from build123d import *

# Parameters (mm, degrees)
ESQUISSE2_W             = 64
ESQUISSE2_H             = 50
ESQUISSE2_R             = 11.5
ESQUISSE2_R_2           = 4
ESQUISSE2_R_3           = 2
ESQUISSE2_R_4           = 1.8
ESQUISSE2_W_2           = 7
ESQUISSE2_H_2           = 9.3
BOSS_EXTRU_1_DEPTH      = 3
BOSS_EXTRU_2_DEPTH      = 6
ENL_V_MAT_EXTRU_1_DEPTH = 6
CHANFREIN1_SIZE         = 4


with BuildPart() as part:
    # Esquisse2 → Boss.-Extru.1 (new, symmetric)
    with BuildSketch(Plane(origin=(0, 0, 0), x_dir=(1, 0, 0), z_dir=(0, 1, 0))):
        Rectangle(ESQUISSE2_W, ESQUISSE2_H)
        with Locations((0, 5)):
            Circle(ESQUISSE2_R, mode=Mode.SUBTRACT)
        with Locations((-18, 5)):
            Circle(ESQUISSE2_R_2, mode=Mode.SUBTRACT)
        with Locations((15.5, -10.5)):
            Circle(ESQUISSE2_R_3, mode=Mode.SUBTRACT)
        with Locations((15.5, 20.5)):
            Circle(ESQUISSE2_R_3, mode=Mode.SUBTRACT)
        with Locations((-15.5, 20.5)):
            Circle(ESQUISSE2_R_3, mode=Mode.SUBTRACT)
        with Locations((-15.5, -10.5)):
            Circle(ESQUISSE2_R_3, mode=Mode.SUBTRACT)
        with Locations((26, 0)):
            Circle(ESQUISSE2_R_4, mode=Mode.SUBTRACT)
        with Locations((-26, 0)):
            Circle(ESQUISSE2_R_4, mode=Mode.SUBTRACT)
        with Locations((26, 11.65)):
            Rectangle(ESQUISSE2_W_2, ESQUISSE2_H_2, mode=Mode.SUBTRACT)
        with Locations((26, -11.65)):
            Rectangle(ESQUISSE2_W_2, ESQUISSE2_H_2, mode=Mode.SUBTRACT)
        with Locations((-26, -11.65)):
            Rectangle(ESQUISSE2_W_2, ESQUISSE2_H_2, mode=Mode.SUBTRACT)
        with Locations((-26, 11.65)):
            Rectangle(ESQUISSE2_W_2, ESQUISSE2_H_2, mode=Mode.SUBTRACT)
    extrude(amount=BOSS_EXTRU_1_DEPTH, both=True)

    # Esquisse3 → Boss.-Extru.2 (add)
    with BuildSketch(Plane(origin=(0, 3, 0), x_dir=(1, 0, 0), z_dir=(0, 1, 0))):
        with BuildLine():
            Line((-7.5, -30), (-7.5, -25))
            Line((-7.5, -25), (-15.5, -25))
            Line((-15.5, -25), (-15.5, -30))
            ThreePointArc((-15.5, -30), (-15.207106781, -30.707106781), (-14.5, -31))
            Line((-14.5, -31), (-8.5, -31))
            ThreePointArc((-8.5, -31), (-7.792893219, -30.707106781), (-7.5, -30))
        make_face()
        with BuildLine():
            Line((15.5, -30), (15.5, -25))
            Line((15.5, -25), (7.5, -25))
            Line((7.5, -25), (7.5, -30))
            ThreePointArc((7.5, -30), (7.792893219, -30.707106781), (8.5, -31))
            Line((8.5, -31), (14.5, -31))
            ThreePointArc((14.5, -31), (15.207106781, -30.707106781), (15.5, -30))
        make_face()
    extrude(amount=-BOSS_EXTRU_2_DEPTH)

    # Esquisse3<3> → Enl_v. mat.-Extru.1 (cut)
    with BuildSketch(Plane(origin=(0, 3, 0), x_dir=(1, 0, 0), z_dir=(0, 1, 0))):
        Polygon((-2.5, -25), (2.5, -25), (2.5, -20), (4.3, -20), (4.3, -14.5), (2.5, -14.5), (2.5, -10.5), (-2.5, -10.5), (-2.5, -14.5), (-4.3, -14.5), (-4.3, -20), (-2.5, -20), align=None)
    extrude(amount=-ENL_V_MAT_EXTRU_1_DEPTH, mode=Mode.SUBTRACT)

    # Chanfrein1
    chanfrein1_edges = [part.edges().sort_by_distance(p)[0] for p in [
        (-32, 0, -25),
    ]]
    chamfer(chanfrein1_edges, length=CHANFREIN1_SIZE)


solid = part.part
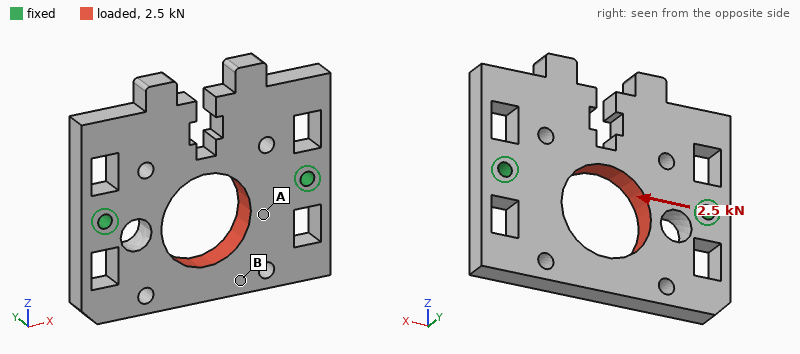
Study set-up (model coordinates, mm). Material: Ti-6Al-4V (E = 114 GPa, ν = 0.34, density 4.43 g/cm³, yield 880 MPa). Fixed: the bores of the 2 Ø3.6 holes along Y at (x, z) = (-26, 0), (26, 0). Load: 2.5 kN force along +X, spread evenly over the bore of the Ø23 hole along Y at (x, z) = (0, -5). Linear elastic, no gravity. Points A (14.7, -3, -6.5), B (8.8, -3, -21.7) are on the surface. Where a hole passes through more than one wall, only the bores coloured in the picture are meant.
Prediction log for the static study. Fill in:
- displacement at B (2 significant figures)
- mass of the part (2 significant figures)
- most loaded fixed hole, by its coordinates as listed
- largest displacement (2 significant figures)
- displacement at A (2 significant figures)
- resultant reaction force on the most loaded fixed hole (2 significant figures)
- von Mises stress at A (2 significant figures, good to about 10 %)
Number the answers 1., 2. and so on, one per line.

1. 7.8 µm
2. 64 g
3. (26, 0)
4. 8.5 µm
5. 3.4 µm
6. 1.4 kN
7. 18 MPa
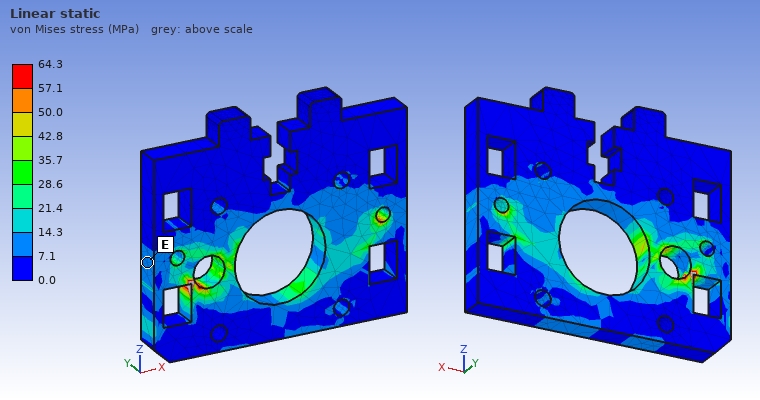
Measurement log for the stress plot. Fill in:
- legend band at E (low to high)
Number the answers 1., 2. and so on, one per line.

1. 7.1 to 14.3 MPa
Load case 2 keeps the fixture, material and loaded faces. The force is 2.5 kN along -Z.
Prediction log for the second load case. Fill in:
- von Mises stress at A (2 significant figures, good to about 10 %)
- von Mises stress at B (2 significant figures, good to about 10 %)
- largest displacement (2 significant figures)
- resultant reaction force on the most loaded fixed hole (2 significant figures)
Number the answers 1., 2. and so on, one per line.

1. 16 MPa
2. 11 MPa
3. 14 µm
4. 1.3 kN
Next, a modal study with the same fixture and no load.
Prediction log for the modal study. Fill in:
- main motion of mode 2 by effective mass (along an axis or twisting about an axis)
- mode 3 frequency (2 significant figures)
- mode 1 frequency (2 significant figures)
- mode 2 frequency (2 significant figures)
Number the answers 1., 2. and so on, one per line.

1. along Y
2. 5400 Hz
3. 3600 Hz
4. 4700 Hz
